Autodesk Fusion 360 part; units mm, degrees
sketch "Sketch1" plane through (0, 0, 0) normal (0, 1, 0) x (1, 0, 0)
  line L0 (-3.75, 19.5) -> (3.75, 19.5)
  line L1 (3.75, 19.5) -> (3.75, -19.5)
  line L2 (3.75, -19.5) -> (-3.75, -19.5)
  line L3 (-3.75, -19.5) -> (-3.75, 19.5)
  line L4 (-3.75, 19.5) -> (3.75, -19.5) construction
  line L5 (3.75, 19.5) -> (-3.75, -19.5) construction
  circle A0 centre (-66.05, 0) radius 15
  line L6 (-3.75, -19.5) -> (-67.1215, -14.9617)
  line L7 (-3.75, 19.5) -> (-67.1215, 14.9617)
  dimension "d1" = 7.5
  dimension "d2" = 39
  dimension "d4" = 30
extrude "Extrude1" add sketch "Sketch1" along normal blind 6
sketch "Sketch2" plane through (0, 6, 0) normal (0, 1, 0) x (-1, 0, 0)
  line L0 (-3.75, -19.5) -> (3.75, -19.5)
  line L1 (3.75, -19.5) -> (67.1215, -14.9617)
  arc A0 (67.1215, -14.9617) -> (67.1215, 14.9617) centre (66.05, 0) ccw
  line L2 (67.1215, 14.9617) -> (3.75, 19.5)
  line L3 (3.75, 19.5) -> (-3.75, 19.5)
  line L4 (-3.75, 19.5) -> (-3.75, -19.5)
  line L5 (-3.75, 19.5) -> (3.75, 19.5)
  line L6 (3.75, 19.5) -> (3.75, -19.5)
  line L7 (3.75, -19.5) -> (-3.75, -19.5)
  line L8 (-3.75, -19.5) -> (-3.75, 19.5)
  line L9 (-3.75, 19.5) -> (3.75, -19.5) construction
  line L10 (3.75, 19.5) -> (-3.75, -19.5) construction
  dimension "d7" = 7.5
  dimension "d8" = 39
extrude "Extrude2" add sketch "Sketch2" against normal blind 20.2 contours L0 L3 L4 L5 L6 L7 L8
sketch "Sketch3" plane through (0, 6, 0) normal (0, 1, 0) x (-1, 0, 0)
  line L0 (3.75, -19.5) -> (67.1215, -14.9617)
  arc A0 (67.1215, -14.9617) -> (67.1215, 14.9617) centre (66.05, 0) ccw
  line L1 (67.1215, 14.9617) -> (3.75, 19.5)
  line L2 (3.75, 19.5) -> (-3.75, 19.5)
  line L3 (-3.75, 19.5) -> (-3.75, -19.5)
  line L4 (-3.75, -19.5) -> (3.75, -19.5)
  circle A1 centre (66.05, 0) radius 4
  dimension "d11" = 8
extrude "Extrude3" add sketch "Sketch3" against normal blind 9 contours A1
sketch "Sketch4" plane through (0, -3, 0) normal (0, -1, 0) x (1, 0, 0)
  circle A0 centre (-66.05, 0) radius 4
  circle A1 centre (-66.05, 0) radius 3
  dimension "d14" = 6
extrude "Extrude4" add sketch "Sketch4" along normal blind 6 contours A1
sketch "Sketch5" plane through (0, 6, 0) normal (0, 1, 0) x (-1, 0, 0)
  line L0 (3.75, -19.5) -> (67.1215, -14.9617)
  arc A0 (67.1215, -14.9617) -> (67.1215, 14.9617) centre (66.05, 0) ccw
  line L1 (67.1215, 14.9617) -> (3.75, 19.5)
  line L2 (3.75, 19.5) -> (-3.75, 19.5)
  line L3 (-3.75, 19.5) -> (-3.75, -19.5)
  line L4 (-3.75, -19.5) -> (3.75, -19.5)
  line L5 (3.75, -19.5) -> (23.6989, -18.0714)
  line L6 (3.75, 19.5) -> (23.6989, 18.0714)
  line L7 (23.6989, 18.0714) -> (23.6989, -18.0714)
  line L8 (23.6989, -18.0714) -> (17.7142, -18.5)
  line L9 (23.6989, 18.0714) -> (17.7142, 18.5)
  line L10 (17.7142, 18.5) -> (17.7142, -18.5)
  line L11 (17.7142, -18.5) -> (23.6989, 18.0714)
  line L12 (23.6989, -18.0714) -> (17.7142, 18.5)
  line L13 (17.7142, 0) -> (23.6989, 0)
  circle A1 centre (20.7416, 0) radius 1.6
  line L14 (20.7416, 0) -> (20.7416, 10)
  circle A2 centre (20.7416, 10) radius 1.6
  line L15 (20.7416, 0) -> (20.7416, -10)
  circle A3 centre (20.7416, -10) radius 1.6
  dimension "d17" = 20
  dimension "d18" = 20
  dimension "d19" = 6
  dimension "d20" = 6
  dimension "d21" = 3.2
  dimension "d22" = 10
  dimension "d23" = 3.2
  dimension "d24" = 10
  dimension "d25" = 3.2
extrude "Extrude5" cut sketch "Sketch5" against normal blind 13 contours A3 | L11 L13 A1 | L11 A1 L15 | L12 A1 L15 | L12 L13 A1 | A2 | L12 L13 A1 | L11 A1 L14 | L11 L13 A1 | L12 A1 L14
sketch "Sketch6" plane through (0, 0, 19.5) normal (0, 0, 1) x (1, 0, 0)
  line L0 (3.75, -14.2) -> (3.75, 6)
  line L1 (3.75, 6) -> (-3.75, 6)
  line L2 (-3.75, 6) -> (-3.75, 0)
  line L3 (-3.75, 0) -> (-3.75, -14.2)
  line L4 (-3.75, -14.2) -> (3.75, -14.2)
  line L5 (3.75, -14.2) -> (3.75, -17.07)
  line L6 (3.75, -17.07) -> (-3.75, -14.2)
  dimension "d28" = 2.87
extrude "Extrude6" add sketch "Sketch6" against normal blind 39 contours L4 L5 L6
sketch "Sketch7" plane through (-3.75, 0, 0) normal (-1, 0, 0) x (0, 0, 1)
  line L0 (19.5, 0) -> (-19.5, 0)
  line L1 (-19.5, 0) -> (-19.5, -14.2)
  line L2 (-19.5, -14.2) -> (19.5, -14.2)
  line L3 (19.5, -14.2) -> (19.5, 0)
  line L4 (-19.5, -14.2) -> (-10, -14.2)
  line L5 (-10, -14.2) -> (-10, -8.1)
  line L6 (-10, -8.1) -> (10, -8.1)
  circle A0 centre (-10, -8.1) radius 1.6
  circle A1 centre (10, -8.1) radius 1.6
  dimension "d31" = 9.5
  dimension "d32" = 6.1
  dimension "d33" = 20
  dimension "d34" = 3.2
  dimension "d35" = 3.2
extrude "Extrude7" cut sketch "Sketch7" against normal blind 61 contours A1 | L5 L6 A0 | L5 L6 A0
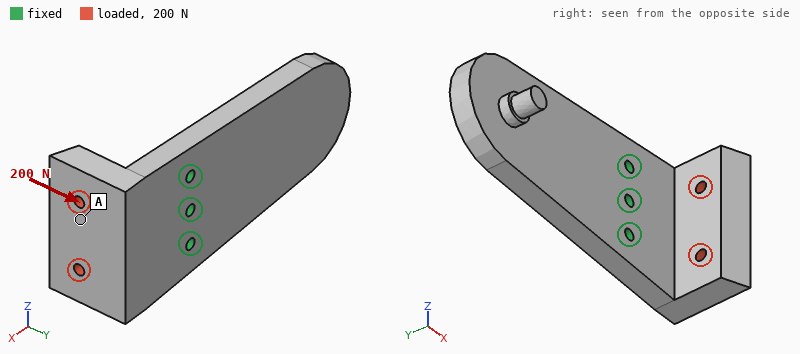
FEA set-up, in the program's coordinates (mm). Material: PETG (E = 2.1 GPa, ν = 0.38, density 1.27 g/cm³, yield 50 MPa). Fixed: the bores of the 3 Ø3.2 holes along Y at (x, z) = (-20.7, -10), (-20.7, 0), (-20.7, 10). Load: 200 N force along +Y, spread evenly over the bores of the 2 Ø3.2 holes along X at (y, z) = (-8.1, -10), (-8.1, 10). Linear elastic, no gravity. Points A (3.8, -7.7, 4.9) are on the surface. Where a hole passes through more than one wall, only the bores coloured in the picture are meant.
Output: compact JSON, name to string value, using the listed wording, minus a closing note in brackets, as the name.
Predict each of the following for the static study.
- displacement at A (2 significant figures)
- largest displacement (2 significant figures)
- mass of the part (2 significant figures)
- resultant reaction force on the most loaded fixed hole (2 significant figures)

{"displacement at A": "0.62 mm", "largest displacement": "0.79 mm", "mass of the part": "27 g", "resultant reaction force on the most loaded fixed hole": "71 N"}
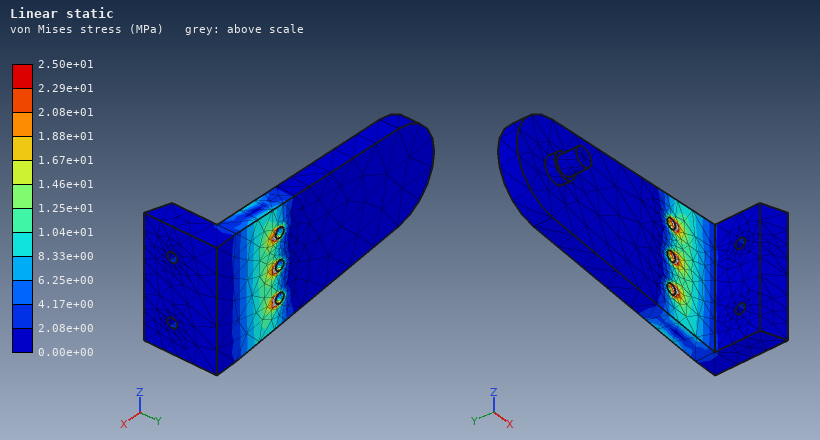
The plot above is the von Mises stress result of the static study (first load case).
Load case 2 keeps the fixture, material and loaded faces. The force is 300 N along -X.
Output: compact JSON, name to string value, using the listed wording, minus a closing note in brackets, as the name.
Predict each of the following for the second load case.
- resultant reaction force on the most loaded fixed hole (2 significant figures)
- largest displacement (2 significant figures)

{"resultant reaction force on the most loaded fixed hole": "110 N", "largest displacement": "1.1 mm"}
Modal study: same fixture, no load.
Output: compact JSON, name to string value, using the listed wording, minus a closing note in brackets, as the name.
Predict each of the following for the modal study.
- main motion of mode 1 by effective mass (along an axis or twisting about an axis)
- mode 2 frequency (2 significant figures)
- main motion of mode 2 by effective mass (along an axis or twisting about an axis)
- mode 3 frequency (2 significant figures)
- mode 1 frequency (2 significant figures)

{"main motion of mode 1 by effective mass": "along Y", "mode 2 frequency": "960 Hz", "main motion of mode 2 by effective mass": "along Y", "mode 3 frequency": "1500 Hz", "mode 1 frequency": "400 Hz"}
